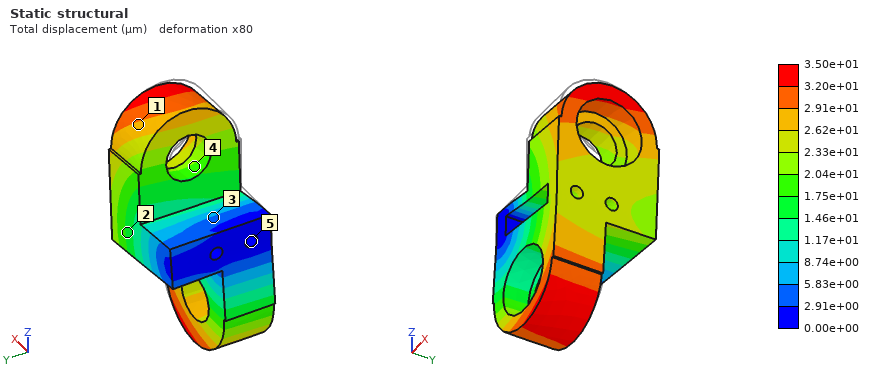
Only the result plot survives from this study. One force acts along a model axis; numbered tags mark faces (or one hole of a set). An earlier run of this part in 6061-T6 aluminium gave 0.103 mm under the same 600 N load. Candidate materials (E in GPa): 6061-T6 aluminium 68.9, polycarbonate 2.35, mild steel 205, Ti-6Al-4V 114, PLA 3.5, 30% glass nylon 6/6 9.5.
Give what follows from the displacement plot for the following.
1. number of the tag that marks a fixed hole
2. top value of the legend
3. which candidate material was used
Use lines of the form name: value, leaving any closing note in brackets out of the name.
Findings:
number of the tag that marks a fixed hole: 5
top value of the legend: 3.50e+01 µm
which candidate material was used: mild steel
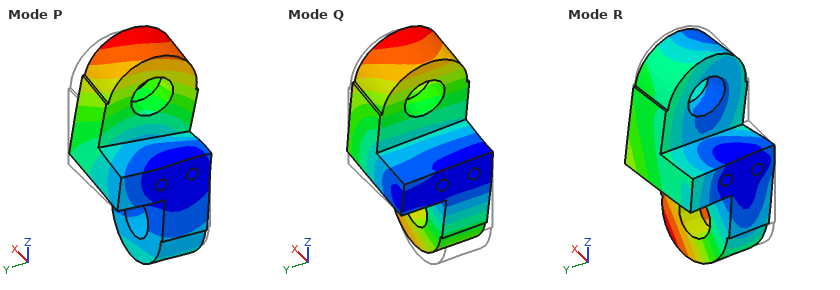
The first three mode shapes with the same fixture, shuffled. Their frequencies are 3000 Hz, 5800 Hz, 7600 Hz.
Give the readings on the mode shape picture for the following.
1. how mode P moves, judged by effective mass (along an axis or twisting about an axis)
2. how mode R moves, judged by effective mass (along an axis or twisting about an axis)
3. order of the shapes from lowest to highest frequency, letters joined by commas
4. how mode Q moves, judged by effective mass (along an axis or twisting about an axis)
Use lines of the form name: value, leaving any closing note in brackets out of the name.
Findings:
how mode P moves, judged by effective mass: along Y
how mode R moves, judged by effective mass: along Y
order of the shapes from lowest to highest frequency, letters joined by commas: Q, P, R
how mode Q moves, judged by effective mass: along Z
